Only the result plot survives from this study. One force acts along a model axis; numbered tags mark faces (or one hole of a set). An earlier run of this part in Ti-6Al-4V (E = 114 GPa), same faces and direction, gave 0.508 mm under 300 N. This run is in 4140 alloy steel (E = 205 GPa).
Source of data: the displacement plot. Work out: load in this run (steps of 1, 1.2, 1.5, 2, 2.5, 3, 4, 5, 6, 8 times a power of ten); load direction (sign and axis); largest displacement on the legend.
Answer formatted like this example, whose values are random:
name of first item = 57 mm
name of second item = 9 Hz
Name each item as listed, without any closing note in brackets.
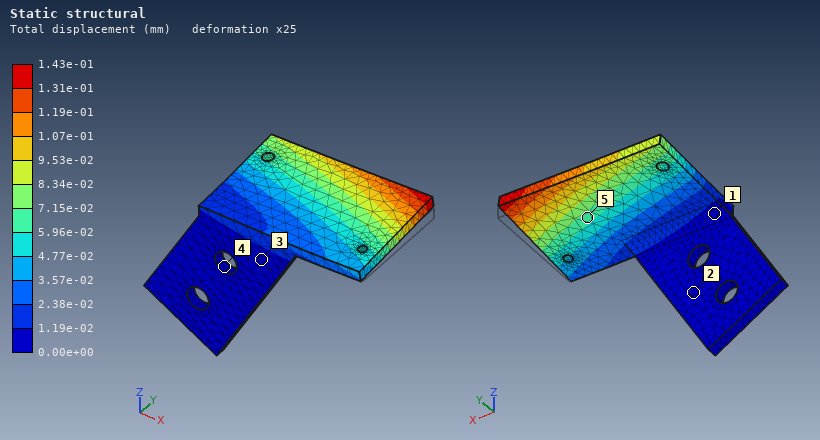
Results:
load in this run = 150 N
load direction = +Z
largest displacement on the legend = 1.43e-01 mm
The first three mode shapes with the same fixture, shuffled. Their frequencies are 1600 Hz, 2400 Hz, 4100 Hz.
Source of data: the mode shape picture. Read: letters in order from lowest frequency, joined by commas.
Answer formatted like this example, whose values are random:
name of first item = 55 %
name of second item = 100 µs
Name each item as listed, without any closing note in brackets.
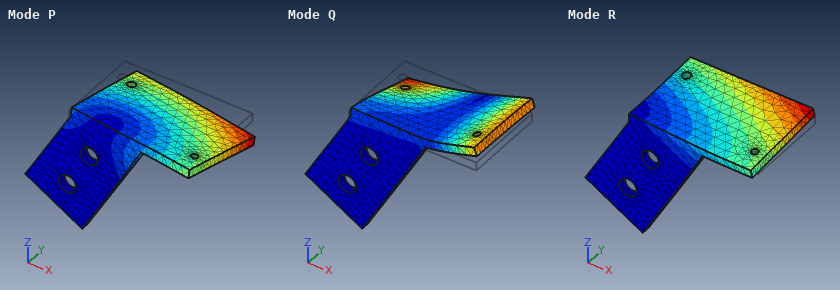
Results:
letters in order from lowest frequency, joined by commas = R, P, Q
